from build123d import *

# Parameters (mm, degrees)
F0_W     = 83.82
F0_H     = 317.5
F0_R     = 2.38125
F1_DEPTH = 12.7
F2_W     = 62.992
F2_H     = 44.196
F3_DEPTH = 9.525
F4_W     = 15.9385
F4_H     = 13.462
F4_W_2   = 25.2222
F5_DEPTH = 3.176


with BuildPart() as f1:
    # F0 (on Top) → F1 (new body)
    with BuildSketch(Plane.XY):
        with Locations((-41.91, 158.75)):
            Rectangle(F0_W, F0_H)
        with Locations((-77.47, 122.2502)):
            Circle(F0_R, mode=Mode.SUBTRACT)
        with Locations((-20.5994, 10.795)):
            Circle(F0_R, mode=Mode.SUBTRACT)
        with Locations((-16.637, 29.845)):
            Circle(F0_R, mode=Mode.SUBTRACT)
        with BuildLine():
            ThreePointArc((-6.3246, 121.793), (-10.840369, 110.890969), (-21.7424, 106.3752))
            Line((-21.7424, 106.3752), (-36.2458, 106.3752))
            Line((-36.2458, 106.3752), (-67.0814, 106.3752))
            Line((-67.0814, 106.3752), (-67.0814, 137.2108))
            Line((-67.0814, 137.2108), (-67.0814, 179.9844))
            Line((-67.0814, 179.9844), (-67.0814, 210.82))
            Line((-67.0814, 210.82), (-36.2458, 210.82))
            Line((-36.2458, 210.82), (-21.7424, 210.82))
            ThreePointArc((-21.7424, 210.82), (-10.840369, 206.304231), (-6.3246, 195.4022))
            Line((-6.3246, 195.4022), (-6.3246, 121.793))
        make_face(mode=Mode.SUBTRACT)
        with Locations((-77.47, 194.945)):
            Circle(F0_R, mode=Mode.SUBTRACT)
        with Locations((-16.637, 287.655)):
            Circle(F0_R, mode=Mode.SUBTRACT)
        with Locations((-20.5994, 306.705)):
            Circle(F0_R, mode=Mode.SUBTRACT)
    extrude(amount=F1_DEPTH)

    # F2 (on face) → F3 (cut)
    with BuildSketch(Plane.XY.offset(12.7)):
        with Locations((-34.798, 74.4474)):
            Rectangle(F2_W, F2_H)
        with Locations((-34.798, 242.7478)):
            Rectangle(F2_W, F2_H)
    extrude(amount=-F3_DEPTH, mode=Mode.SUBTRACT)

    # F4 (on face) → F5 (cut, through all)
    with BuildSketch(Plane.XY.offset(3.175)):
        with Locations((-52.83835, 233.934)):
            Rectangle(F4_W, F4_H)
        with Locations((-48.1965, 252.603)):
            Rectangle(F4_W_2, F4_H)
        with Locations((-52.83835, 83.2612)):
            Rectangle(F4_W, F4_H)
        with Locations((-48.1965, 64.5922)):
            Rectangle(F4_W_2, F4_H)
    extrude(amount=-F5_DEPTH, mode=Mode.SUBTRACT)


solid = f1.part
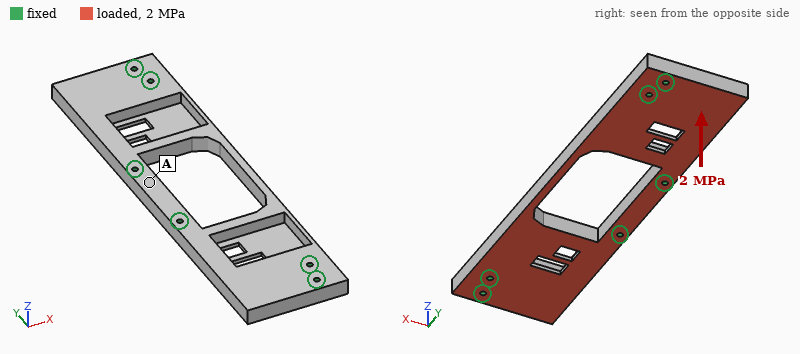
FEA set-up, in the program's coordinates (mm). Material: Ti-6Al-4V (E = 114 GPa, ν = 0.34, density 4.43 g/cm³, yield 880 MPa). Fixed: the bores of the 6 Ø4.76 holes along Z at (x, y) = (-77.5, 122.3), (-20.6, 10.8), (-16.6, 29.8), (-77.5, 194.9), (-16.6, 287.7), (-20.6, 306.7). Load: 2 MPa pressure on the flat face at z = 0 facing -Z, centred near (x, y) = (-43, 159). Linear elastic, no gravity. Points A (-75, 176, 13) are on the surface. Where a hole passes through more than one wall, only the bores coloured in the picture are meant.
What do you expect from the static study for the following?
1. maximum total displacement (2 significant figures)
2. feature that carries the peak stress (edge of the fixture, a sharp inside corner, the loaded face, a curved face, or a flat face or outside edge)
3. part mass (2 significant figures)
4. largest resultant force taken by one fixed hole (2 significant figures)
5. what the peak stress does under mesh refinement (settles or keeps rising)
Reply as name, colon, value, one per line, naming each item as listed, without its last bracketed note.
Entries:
maximum total displacement: 0.78 mm
feature that carries the peak stress: edge of the fixture
part mass: 890 g
largest resultant force taken by one fixed hole: 12 kN
what the peak stress does under mesh refinement: keeps rising
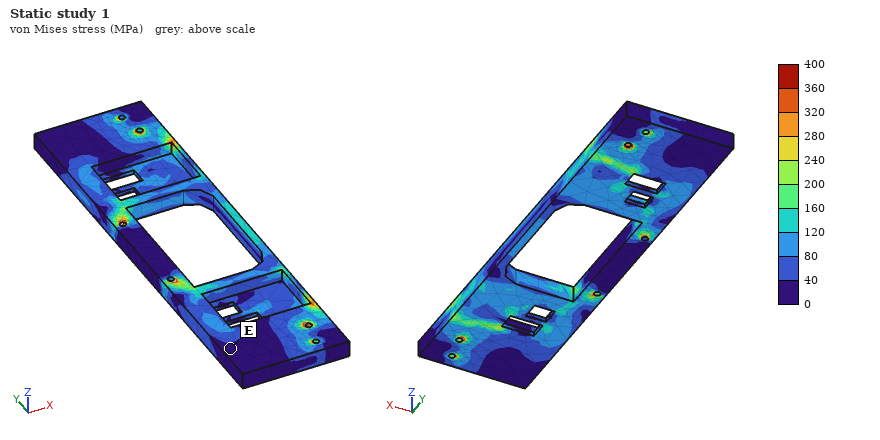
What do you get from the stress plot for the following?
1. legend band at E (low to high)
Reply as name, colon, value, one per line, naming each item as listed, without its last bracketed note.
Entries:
legend band at E: 0 to 40 MPa
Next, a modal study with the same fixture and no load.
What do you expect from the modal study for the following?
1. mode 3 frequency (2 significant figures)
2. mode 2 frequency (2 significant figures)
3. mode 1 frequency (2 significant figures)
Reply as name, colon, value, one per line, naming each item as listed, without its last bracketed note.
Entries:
mode 3 frequency: 2500 Hz
mode 2 frequency: 2400 Hz
mode 1 frequency: 1500 Hz
